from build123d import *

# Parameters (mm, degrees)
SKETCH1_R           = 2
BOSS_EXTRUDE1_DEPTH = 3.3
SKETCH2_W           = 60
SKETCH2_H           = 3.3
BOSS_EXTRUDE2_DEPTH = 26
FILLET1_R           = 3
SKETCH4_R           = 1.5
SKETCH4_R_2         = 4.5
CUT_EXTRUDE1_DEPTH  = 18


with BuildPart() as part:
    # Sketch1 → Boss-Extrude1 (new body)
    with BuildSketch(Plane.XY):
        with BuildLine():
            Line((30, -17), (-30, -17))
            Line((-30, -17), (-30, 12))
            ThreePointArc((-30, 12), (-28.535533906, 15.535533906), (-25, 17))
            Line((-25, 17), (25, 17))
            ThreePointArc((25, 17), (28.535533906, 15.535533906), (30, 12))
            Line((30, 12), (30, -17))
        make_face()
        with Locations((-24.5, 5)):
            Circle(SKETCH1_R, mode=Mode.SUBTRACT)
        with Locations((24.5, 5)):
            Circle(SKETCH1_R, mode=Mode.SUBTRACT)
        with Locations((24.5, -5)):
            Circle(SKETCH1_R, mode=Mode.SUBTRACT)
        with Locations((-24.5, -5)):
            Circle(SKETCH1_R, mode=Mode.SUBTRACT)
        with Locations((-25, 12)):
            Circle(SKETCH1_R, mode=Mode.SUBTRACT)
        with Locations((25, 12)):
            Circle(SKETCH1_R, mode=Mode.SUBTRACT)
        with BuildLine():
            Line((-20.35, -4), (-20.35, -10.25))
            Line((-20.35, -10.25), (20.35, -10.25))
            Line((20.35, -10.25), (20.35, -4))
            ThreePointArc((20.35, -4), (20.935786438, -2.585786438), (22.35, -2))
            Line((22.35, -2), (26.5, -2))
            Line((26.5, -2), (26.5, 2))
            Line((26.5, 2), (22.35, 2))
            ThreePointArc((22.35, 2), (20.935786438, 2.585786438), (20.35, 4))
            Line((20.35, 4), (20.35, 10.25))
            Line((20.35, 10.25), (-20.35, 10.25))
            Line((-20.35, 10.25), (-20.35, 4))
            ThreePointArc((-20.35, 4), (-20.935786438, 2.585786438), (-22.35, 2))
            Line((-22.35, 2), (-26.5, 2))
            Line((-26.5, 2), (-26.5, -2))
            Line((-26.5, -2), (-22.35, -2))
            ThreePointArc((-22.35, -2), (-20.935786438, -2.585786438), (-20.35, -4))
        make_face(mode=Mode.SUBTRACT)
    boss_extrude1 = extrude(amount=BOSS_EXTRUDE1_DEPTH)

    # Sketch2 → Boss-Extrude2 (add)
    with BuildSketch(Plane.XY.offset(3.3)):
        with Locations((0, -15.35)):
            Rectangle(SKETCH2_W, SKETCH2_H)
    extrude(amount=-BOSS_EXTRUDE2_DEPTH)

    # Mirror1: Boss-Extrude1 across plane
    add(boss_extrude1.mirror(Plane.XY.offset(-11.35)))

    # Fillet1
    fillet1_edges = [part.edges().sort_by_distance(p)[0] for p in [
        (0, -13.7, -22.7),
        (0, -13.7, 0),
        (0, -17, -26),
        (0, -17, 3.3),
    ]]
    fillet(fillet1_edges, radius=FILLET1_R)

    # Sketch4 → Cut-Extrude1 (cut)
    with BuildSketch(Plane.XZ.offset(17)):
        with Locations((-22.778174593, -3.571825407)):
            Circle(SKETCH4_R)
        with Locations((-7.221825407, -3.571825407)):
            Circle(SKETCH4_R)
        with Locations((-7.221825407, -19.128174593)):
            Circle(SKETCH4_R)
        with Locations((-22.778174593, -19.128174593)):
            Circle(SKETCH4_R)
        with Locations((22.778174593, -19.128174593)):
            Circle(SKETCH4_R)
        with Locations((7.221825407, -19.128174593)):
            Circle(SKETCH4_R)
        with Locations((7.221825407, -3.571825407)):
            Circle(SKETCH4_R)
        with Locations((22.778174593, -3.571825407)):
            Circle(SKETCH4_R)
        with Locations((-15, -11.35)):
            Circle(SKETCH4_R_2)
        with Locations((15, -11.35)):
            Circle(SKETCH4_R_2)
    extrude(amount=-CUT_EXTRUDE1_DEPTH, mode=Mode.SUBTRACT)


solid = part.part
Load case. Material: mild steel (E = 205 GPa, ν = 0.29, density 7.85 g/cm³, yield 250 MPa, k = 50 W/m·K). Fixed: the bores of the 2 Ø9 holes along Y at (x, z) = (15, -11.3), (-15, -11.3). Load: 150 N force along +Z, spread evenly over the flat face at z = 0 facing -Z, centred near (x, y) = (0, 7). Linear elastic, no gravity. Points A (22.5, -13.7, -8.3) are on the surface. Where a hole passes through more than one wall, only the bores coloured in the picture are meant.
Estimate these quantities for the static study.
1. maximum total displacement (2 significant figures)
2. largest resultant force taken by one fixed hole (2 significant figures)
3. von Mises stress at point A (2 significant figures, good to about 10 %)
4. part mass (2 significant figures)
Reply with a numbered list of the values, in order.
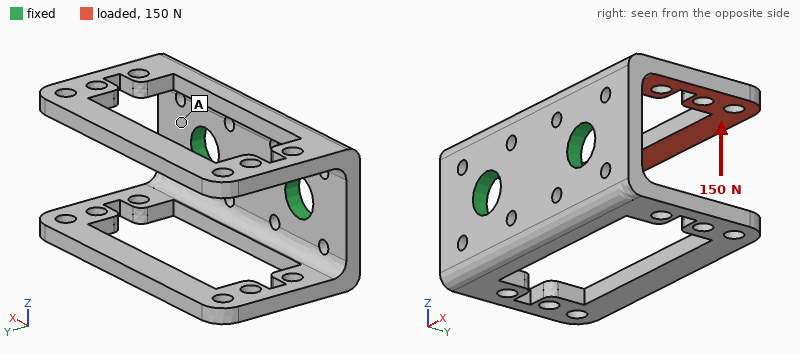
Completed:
1. 0.18 mm
2. 75 N
3. 20 MPa
4. 86 g
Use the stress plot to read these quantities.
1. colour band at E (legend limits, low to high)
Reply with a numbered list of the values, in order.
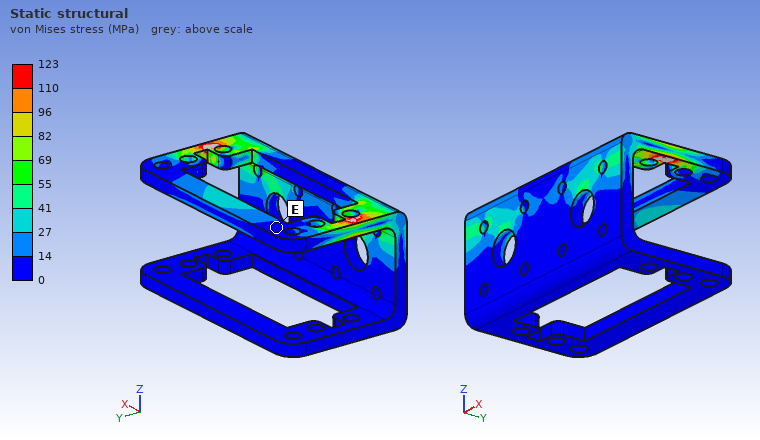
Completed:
1. 0 to 14 MPa
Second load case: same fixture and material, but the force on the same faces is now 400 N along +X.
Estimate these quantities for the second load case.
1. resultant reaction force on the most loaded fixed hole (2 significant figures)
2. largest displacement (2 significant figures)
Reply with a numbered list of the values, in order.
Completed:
1. 290 N
2. 59 µm
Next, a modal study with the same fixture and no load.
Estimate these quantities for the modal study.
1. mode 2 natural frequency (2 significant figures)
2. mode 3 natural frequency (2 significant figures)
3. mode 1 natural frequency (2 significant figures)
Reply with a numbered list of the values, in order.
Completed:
1. 1300 Hz
2. 2700 Hz
3. 1300 Hz
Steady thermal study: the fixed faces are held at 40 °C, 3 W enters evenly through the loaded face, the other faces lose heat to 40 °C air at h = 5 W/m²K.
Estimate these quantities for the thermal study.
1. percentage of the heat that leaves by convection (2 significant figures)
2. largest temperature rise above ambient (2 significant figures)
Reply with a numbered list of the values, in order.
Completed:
1. 9.6 %
2. 43 K
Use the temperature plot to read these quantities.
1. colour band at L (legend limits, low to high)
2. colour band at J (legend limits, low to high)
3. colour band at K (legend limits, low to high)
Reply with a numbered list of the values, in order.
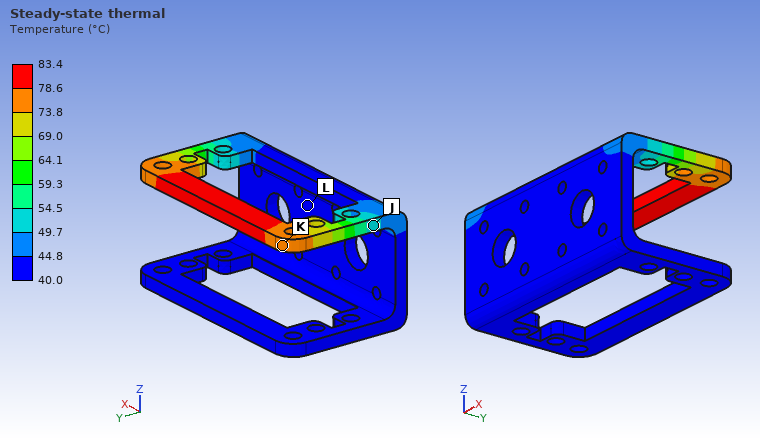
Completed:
1. 40.0 to 44.8 °C
2. 49.7 to 54.5 °C
3. 73.8 to 78.6 °C
